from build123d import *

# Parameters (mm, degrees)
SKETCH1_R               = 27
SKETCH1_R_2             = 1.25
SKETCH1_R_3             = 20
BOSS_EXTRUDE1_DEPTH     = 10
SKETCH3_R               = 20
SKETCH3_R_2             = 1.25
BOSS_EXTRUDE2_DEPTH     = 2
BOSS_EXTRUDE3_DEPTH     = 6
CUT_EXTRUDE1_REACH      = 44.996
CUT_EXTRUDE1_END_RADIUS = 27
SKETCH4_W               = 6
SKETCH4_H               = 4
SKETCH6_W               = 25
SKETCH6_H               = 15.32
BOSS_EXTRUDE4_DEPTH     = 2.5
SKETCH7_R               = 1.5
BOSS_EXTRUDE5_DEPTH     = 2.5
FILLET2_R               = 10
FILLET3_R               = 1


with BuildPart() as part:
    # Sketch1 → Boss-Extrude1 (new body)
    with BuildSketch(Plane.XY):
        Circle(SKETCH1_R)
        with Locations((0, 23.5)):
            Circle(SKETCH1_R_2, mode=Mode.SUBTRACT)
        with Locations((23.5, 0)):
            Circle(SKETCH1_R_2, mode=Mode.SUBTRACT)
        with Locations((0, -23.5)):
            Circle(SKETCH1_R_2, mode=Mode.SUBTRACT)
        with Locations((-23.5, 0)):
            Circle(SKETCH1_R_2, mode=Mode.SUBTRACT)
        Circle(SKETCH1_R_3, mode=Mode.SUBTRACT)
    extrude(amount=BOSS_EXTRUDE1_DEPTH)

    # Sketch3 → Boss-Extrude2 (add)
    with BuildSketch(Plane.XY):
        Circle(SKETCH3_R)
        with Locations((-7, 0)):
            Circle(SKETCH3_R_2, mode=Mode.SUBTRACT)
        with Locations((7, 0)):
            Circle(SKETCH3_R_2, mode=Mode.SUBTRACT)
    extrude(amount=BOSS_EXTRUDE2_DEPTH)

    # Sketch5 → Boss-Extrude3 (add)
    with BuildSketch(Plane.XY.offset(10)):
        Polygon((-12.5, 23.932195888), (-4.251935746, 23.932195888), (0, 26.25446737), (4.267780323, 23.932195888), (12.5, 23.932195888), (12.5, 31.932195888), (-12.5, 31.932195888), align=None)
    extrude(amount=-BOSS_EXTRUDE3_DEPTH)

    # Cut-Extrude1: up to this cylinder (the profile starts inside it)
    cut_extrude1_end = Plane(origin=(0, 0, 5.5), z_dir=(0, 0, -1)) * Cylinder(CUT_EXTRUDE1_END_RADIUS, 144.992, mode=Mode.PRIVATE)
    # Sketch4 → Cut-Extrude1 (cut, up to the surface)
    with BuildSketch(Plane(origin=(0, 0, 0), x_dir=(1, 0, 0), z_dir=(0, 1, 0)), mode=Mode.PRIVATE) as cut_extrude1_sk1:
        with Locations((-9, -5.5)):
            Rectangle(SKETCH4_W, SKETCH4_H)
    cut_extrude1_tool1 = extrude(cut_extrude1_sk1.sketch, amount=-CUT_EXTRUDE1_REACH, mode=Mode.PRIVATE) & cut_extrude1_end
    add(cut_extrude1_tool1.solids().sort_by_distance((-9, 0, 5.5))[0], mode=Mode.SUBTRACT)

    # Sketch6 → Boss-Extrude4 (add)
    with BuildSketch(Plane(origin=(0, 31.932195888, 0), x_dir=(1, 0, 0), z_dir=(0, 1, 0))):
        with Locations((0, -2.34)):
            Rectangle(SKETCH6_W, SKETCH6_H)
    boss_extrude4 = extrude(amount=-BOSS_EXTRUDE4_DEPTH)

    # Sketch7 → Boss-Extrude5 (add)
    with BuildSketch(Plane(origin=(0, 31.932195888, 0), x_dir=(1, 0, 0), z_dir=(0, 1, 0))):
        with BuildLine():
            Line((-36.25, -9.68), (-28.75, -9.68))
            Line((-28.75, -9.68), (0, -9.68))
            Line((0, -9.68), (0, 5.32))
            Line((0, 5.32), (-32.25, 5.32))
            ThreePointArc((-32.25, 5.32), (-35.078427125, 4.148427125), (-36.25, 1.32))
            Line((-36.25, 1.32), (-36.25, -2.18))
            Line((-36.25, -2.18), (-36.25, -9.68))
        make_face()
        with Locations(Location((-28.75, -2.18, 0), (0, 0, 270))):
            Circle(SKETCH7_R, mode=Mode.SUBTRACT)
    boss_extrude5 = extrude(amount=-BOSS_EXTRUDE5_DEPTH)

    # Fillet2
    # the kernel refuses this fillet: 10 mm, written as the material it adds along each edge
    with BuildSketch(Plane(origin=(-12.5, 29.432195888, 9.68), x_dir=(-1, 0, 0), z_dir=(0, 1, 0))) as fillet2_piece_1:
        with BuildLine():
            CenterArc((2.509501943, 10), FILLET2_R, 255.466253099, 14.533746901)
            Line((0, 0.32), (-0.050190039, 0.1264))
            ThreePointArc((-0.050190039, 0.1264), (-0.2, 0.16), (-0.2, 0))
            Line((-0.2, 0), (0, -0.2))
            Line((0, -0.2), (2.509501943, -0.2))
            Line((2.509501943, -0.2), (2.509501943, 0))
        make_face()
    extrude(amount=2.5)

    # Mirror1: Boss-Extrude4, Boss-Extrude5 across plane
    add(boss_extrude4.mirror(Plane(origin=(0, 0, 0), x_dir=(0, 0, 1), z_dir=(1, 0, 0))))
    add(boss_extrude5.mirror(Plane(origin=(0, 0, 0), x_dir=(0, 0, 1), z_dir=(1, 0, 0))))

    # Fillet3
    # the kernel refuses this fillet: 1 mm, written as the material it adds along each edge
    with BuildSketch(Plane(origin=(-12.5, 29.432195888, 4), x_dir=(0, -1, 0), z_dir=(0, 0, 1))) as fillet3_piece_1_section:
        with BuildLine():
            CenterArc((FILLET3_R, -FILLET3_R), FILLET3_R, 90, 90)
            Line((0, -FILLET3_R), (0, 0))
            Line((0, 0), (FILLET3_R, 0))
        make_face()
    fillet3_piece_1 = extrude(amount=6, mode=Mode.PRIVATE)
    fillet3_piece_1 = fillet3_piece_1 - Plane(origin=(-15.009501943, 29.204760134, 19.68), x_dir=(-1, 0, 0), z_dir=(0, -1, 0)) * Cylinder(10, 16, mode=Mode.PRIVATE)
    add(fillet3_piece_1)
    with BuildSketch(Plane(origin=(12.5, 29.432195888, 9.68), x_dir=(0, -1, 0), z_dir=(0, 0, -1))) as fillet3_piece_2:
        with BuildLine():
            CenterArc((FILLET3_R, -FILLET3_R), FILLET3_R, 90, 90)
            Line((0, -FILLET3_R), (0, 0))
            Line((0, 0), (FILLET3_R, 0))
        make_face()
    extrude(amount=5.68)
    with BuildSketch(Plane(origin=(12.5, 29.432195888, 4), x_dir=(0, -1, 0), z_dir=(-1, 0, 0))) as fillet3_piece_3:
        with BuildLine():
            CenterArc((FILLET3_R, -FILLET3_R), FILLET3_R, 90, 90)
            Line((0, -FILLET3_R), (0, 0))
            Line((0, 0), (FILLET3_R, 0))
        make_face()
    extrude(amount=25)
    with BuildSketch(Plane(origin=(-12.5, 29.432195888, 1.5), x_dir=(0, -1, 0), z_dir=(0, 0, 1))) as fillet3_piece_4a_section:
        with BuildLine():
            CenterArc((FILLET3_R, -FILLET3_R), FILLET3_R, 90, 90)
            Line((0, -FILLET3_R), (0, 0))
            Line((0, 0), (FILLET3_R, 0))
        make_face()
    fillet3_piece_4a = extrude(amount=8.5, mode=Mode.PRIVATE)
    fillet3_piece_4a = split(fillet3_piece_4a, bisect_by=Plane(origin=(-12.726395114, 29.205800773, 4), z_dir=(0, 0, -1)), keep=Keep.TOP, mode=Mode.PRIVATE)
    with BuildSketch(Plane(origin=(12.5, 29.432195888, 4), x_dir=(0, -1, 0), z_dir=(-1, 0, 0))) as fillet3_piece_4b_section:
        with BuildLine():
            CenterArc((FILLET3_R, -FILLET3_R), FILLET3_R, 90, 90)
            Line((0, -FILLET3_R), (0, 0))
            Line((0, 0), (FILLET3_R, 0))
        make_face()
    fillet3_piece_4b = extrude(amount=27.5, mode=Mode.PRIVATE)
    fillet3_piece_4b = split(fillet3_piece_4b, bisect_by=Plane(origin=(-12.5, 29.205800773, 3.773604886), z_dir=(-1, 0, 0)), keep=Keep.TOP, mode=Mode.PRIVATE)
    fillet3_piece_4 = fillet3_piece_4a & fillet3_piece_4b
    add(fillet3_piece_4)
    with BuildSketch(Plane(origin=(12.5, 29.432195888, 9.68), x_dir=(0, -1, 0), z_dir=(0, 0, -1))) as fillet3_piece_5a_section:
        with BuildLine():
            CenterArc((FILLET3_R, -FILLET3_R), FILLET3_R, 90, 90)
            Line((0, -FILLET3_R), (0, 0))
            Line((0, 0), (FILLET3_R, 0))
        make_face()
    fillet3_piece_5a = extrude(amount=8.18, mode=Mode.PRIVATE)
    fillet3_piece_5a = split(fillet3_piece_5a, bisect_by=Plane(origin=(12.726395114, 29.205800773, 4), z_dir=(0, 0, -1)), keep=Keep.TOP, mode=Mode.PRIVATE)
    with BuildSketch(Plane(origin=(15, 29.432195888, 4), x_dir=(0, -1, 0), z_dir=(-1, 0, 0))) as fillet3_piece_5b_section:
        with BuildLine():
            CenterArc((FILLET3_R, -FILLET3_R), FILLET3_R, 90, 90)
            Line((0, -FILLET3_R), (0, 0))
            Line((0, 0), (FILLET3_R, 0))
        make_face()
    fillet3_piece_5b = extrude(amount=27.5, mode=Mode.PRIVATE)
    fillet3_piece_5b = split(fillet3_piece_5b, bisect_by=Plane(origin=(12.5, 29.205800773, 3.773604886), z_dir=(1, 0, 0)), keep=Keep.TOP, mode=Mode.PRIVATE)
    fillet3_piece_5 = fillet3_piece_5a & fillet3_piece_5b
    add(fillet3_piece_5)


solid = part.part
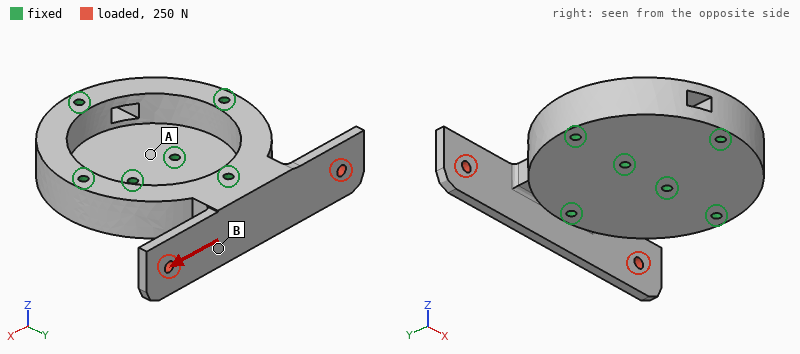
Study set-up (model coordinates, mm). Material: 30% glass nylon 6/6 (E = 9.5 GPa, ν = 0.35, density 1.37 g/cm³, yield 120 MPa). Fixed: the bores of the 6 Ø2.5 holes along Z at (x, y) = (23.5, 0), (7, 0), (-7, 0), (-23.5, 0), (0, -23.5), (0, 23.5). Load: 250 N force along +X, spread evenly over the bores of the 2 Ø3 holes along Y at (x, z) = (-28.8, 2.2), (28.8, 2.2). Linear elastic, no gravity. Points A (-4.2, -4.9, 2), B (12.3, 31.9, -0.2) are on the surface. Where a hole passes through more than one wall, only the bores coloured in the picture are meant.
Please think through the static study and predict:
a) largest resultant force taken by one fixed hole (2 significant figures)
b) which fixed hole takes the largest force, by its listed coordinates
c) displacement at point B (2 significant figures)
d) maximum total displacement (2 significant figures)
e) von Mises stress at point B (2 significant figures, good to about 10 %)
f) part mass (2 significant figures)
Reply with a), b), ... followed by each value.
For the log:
a) 200 N
b) (0, 23.5)
c) 26 µm
d) 64 µm
e) 3.9 MPa
f) 21 g
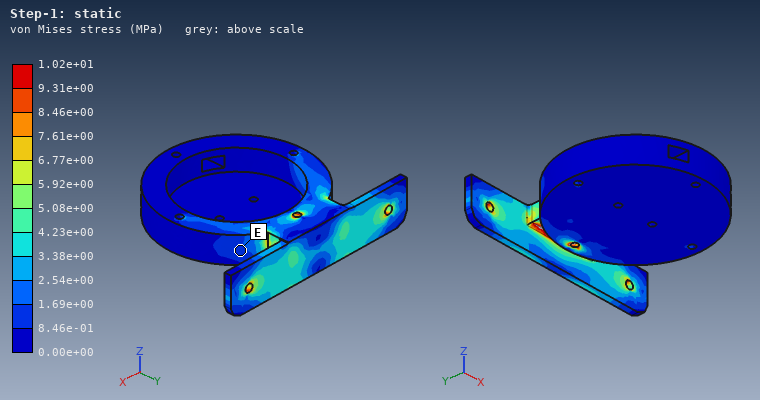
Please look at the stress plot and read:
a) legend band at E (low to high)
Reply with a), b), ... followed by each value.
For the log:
a) 8.46e-01 to 1.69e+00 MPa
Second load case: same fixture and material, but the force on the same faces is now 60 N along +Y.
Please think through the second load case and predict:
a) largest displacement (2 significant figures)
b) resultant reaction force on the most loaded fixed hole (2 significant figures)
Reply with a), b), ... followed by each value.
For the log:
a) 0.58 mm
b) 21 N
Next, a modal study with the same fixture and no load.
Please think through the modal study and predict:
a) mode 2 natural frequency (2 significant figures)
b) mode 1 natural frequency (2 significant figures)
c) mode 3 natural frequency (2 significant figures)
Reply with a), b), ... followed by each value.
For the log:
a) 1600 Hz
b) 1600 Hz
c) 3300 Hz
